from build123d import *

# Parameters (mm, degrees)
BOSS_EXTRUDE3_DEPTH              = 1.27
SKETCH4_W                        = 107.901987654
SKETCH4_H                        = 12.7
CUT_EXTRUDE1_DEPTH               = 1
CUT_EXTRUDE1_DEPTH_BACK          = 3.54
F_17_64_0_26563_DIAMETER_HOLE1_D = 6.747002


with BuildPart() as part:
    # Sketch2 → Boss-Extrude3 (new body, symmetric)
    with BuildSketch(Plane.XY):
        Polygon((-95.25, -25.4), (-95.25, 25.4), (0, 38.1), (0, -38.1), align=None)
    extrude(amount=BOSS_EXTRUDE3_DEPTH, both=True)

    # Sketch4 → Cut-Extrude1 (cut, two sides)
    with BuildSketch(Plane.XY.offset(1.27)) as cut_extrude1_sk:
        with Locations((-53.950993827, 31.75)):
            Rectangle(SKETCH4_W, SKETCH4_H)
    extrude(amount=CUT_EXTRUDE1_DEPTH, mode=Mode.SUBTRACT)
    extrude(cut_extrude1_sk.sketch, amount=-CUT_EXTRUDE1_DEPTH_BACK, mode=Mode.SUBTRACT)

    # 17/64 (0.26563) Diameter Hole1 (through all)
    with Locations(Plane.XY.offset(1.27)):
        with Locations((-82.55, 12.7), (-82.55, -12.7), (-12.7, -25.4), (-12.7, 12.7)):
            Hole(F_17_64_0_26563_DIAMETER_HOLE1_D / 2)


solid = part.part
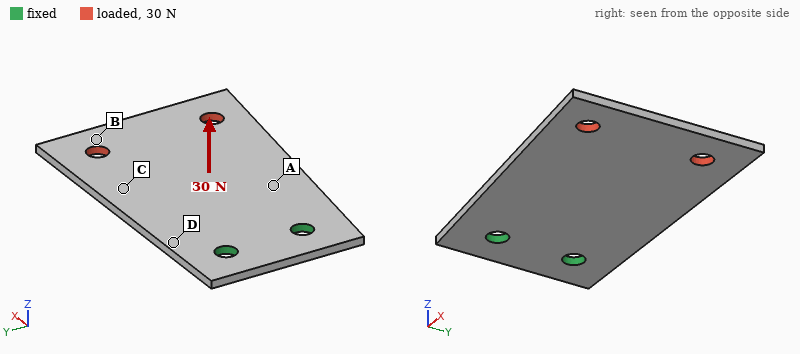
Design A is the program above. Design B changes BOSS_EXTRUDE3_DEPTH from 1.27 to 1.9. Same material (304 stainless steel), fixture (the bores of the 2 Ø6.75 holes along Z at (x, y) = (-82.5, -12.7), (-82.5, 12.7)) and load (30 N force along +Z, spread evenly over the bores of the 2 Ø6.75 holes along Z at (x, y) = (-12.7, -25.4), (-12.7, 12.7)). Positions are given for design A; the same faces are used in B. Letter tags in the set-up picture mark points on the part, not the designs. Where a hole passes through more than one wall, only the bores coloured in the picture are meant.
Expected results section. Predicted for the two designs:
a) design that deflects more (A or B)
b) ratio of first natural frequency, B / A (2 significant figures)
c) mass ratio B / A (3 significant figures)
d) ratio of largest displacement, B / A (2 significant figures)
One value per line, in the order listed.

A
1.5
1.50
0.30
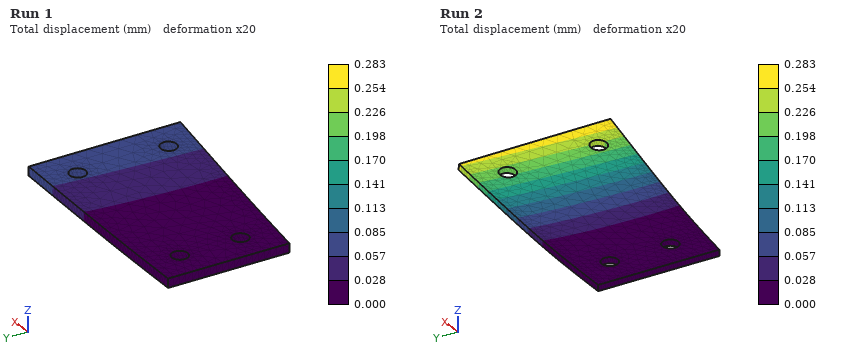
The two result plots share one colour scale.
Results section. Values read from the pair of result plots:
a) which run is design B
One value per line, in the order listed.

Run 1
